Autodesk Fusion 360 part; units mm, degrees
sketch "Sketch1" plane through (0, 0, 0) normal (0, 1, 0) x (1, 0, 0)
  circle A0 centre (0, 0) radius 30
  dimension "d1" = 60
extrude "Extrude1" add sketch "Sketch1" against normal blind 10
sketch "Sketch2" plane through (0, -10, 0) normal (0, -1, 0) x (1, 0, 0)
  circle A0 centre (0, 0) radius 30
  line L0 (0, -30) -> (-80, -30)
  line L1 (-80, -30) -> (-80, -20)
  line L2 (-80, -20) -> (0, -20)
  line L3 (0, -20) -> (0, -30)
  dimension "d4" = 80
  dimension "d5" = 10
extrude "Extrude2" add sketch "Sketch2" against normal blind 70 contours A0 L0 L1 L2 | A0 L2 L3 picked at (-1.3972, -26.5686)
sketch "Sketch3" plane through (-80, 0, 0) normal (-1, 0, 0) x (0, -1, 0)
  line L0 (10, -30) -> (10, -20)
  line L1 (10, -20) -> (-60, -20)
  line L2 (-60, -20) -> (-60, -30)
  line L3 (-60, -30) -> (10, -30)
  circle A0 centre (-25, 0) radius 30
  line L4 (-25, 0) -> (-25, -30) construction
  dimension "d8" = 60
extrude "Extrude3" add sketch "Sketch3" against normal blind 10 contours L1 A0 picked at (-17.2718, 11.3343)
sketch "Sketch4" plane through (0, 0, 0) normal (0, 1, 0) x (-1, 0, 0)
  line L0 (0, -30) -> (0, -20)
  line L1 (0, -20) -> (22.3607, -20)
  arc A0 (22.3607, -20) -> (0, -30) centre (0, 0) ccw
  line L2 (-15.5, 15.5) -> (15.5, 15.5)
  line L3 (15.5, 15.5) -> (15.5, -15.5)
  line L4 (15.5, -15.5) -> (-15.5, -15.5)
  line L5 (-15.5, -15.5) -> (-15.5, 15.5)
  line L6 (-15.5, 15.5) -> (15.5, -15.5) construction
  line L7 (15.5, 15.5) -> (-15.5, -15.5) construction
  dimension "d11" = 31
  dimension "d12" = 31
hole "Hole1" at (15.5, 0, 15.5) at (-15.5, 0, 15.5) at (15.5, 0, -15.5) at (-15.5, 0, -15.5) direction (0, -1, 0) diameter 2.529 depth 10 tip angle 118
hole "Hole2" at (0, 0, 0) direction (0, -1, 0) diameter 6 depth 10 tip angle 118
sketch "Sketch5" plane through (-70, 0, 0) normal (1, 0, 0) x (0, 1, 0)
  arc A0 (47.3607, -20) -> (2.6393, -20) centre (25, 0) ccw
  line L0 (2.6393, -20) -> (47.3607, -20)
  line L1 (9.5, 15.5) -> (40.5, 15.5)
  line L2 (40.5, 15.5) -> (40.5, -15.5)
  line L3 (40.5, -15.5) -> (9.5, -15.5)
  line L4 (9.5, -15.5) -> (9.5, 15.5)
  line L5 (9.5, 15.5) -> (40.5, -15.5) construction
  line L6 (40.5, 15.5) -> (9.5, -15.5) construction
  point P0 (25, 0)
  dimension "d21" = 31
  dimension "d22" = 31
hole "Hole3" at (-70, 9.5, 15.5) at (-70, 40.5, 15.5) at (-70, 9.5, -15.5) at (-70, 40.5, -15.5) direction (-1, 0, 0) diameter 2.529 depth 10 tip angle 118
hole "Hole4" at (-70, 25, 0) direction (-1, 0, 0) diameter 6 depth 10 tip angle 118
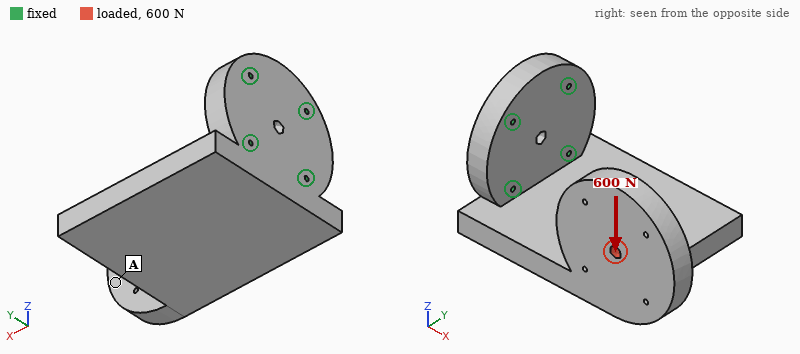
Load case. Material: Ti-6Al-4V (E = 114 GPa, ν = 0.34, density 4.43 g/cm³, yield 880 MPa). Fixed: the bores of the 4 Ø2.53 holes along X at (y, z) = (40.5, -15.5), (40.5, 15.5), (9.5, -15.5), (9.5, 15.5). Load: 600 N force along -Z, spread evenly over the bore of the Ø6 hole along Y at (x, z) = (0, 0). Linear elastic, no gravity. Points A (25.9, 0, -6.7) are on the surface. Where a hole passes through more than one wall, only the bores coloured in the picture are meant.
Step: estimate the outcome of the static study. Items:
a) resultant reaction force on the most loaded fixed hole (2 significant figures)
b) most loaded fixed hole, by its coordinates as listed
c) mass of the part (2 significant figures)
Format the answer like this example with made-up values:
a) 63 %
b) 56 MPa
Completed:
a) 790 N
b) (9.5, -15.5)
c) 470 g
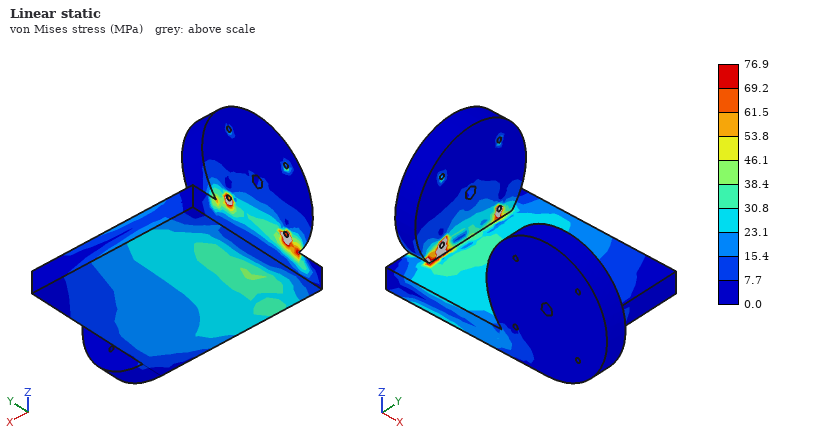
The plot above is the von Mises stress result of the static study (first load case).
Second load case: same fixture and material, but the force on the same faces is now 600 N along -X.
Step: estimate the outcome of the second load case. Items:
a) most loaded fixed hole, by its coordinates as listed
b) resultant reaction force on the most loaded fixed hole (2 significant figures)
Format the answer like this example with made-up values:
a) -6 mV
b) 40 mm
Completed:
a) (9.5, -15.5)
b) 750 N
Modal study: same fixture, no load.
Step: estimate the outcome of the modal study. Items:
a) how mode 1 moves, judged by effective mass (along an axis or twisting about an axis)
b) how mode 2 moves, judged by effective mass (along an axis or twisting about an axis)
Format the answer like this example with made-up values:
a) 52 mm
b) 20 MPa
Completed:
a) along Z
b) along Y
